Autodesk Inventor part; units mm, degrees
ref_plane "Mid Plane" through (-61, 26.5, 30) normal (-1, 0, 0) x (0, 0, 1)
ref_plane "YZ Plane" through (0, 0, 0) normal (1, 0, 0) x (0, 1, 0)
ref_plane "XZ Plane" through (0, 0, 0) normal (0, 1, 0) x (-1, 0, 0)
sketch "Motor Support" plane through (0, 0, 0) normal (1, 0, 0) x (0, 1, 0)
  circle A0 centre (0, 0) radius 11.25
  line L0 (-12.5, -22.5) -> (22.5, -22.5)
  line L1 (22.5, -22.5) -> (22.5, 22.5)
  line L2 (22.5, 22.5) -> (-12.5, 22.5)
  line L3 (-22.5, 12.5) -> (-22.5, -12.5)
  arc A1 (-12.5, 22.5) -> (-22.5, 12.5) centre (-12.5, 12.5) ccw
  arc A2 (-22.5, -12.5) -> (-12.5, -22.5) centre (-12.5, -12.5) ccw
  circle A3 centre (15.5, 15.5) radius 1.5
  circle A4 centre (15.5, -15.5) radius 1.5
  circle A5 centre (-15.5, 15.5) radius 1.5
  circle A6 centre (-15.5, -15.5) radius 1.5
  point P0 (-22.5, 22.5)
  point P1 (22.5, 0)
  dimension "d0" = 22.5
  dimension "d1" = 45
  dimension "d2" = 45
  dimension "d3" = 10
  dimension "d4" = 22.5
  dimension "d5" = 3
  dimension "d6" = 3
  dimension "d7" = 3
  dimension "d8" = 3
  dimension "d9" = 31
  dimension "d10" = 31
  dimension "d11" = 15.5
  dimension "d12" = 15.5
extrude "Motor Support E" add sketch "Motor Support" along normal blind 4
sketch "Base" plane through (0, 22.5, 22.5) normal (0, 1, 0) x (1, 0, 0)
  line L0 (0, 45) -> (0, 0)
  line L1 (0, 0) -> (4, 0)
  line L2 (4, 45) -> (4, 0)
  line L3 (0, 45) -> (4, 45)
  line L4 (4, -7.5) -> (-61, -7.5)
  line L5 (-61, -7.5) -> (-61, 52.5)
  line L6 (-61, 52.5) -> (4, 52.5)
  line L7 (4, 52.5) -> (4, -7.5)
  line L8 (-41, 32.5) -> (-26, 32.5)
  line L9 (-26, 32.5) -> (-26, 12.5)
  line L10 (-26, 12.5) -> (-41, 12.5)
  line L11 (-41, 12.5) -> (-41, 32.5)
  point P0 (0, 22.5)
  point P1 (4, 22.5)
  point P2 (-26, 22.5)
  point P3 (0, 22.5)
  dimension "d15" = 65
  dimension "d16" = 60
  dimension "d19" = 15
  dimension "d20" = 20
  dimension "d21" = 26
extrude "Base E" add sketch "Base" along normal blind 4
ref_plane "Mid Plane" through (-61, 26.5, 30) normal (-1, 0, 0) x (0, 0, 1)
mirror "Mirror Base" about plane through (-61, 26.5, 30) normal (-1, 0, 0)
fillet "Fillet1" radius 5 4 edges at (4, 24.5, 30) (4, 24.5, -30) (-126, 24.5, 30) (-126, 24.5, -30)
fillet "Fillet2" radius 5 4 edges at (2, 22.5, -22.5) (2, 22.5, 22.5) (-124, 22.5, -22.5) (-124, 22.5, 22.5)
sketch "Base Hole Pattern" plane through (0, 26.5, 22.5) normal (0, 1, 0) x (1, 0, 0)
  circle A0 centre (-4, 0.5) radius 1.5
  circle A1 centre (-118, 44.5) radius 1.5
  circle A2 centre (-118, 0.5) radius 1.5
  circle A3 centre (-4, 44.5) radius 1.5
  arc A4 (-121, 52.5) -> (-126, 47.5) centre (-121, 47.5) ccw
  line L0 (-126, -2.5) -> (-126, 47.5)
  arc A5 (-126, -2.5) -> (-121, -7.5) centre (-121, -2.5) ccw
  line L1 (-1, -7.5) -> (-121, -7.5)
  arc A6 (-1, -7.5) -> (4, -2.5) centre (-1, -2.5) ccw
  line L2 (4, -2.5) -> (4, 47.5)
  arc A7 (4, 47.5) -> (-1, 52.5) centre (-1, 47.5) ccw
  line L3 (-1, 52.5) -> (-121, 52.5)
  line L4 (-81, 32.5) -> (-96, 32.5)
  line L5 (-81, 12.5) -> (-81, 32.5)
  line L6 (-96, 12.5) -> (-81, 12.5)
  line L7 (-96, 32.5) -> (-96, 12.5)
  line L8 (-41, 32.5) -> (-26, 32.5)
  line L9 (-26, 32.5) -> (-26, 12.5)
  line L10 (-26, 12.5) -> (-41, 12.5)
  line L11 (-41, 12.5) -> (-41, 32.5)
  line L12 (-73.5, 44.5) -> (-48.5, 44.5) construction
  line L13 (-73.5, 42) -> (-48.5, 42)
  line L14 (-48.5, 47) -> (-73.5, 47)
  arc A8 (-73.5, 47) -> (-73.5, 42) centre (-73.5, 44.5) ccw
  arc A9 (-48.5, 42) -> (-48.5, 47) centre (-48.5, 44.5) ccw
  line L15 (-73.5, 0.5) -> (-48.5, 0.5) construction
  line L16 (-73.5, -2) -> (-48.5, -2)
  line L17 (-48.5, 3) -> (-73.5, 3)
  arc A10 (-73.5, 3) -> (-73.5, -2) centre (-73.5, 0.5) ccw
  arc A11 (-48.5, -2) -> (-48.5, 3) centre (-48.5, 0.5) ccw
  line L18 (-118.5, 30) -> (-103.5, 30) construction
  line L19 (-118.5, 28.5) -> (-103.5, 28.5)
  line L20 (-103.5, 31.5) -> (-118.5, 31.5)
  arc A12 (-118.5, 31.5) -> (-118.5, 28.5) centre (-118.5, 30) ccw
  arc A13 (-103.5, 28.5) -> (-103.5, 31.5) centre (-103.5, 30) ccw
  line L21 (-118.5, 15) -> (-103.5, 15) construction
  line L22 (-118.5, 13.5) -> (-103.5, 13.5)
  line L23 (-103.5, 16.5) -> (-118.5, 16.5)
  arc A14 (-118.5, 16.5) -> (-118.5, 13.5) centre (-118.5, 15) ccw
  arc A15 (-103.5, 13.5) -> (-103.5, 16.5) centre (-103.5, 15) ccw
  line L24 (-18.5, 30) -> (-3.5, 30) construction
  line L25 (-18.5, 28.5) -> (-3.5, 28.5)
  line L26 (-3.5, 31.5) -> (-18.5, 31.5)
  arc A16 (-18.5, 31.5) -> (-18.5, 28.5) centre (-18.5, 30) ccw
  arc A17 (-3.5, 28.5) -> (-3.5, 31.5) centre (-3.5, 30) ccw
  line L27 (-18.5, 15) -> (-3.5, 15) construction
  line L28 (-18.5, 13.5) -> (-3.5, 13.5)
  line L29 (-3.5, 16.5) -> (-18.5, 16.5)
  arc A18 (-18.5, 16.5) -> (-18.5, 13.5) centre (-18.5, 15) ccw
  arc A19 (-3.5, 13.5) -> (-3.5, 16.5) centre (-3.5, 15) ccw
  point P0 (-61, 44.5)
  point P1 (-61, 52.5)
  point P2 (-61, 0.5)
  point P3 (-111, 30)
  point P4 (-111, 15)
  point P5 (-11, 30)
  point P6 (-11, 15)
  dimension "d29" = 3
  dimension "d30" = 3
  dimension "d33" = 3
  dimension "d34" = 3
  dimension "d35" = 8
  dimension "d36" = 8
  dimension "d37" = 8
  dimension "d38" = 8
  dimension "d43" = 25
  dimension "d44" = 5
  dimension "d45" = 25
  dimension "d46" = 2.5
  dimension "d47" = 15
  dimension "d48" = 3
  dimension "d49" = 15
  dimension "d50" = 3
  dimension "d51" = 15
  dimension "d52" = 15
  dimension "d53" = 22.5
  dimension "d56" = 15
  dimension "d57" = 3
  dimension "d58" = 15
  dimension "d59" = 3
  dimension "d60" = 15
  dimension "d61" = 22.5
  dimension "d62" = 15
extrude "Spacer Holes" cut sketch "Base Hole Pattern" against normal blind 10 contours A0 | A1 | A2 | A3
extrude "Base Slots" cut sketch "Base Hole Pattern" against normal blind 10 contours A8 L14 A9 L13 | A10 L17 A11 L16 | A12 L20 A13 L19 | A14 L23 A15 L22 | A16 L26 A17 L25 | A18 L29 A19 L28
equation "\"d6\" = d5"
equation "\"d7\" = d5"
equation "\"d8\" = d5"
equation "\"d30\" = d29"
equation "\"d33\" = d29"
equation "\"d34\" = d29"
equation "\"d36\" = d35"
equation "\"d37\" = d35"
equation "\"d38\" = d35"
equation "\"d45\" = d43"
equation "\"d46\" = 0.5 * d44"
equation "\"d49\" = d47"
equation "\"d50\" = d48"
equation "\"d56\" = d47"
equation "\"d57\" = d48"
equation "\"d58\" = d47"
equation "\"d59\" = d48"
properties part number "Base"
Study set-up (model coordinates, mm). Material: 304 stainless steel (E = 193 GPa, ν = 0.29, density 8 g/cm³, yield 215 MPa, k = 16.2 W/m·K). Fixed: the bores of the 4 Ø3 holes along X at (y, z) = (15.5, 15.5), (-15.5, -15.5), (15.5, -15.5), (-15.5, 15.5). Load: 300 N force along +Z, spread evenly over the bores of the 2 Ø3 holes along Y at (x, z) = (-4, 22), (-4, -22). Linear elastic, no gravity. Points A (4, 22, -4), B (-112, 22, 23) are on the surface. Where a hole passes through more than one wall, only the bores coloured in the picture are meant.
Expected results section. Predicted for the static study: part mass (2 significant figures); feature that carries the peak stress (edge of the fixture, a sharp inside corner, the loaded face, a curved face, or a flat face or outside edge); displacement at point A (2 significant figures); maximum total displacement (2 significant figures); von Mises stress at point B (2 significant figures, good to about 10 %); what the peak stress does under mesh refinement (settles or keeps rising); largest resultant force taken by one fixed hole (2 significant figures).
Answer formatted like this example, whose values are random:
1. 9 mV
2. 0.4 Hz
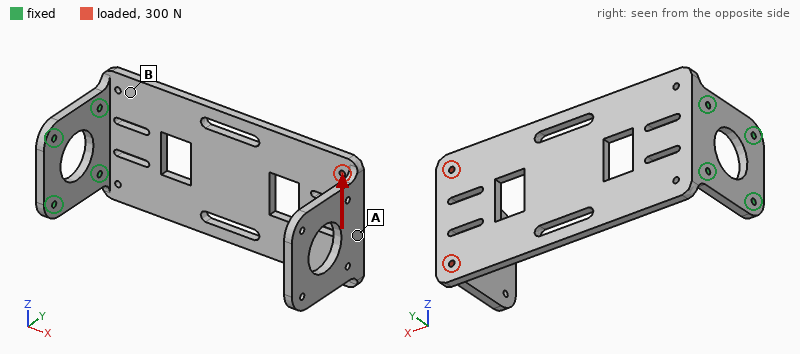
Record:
1. 310 g
2. edge of the fixture
3. 0.13 mm
4. 0.17 mm
5. 29 MPa
6. keeps rising
7. 1.1 kN
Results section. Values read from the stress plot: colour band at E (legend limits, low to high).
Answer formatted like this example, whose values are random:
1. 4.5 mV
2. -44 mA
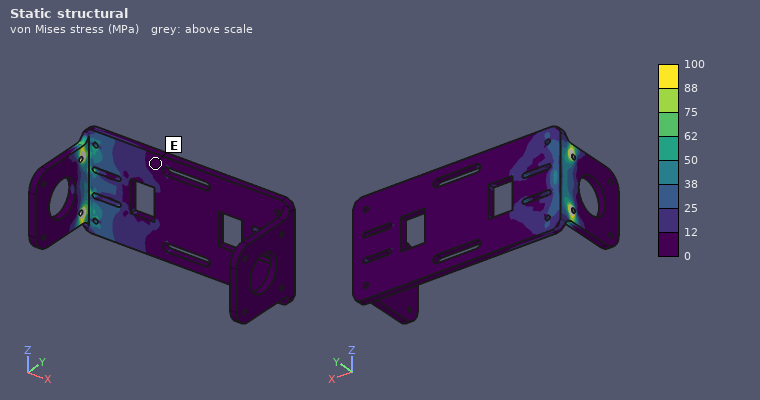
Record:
1. 0 to 12 MPa
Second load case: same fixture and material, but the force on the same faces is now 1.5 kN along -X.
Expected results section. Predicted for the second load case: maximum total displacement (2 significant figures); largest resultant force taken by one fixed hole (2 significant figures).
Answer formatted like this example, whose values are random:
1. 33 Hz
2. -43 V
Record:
1. 0.23 mm
2. 790 N
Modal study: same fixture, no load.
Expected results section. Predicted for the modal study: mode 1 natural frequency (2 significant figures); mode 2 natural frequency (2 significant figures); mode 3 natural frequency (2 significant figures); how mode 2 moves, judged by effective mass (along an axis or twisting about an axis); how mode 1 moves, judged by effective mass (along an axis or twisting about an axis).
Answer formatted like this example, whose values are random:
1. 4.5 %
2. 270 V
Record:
1. 120 Hz
2. 410 Hz
3. 620 Hz
4. along Z
5. along Y
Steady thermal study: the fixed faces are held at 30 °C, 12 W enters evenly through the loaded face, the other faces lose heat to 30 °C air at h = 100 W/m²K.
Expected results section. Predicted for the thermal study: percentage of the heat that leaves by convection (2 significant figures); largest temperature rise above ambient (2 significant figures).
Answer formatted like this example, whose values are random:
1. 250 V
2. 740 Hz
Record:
1. 100 %
2. 53 K
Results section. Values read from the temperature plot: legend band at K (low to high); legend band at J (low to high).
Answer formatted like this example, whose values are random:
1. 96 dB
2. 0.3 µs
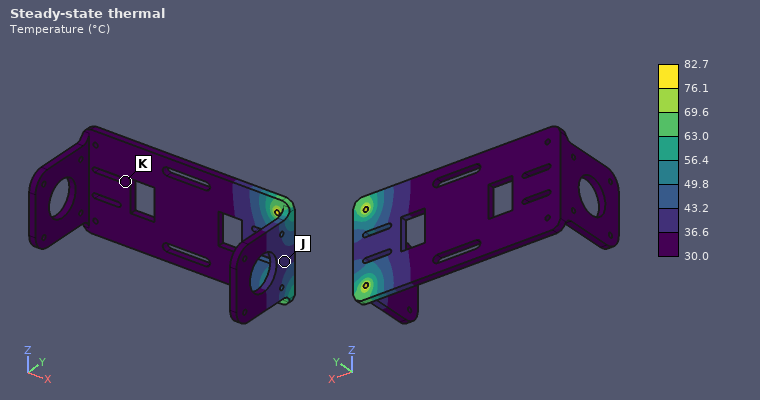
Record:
1. 30.0 to 36.6 °C
2. 36.6 to 43.2 °C
